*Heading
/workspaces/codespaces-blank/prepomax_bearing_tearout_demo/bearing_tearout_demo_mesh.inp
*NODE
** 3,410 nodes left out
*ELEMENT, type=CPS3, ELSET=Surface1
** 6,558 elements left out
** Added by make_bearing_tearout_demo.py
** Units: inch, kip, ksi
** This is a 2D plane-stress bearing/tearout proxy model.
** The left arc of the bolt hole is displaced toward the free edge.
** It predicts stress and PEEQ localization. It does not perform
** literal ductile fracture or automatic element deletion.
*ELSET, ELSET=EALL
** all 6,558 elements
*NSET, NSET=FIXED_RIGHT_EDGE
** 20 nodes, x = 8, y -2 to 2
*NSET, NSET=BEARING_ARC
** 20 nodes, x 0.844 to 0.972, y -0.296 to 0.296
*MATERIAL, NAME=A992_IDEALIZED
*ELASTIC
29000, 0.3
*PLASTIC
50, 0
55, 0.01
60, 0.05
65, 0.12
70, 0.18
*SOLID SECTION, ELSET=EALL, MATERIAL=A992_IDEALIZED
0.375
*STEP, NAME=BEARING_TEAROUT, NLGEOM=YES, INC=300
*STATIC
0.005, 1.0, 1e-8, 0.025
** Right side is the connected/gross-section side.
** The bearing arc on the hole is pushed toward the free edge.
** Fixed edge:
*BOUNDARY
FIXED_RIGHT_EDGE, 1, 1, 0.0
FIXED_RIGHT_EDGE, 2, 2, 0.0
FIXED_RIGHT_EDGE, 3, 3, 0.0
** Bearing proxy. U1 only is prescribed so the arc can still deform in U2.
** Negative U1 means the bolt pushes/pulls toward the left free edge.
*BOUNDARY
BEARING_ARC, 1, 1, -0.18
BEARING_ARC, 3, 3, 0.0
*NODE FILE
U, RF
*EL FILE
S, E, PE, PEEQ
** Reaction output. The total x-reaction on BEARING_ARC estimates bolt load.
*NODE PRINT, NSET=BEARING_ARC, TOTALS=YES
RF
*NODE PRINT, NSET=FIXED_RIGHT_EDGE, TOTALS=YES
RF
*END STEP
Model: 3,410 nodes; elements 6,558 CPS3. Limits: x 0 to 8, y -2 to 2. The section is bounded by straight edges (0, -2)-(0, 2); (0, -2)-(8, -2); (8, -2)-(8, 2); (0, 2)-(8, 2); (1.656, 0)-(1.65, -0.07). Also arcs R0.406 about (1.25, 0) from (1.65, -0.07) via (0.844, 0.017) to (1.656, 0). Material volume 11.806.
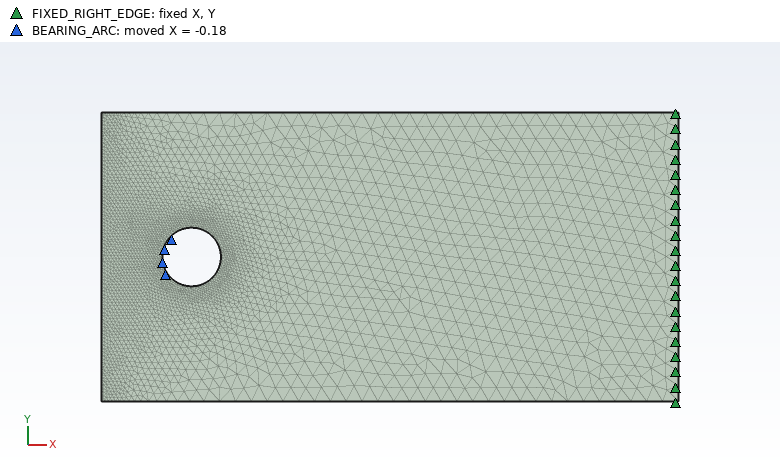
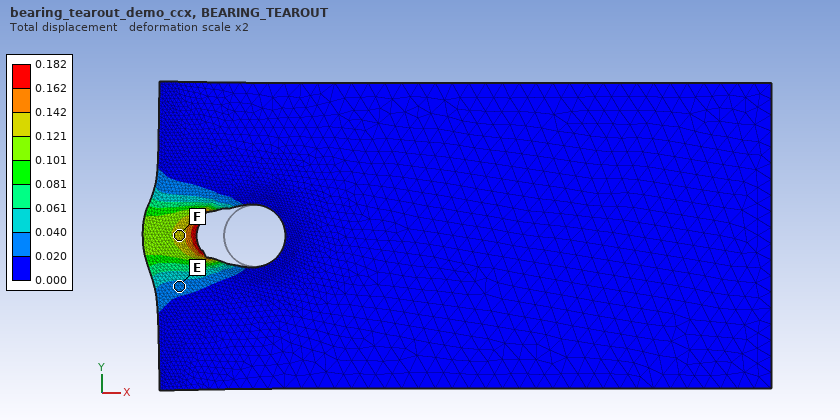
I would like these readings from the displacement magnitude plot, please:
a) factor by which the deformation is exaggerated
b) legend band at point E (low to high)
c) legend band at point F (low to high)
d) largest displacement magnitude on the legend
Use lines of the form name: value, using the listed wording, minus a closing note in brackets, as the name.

factor by which the deformation is exaggerated: 2
legend band at point E: 0.020 to 0.040
legend band at point F: 0.121 to 0.142
largest displacement magnitude on the legend: 0.182
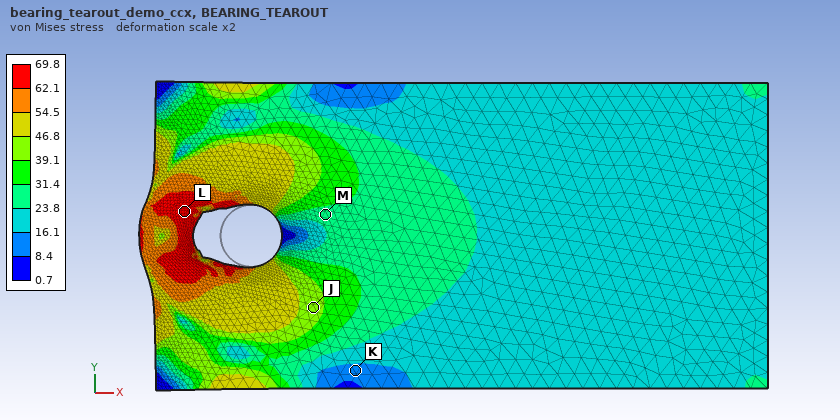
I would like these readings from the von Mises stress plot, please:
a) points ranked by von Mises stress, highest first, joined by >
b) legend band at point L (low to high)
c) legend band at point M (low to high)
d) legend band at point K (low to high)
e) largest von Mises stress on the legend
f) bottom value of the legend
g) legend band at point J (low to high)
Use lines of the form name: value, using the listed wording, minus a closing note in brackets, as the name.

points ranked by von Mises stress, highest first, joined by >: L > J > M > K
legend band at point L: 62.1 to 69.8
legend band at point M: 23.8 to 31.4
legend band at point K: 8.4 to 16.1
largest von Mises stress on the legend: 69.8
bottom value of the legend: 0.7
legend band at point J: 39.1 to 46.8
